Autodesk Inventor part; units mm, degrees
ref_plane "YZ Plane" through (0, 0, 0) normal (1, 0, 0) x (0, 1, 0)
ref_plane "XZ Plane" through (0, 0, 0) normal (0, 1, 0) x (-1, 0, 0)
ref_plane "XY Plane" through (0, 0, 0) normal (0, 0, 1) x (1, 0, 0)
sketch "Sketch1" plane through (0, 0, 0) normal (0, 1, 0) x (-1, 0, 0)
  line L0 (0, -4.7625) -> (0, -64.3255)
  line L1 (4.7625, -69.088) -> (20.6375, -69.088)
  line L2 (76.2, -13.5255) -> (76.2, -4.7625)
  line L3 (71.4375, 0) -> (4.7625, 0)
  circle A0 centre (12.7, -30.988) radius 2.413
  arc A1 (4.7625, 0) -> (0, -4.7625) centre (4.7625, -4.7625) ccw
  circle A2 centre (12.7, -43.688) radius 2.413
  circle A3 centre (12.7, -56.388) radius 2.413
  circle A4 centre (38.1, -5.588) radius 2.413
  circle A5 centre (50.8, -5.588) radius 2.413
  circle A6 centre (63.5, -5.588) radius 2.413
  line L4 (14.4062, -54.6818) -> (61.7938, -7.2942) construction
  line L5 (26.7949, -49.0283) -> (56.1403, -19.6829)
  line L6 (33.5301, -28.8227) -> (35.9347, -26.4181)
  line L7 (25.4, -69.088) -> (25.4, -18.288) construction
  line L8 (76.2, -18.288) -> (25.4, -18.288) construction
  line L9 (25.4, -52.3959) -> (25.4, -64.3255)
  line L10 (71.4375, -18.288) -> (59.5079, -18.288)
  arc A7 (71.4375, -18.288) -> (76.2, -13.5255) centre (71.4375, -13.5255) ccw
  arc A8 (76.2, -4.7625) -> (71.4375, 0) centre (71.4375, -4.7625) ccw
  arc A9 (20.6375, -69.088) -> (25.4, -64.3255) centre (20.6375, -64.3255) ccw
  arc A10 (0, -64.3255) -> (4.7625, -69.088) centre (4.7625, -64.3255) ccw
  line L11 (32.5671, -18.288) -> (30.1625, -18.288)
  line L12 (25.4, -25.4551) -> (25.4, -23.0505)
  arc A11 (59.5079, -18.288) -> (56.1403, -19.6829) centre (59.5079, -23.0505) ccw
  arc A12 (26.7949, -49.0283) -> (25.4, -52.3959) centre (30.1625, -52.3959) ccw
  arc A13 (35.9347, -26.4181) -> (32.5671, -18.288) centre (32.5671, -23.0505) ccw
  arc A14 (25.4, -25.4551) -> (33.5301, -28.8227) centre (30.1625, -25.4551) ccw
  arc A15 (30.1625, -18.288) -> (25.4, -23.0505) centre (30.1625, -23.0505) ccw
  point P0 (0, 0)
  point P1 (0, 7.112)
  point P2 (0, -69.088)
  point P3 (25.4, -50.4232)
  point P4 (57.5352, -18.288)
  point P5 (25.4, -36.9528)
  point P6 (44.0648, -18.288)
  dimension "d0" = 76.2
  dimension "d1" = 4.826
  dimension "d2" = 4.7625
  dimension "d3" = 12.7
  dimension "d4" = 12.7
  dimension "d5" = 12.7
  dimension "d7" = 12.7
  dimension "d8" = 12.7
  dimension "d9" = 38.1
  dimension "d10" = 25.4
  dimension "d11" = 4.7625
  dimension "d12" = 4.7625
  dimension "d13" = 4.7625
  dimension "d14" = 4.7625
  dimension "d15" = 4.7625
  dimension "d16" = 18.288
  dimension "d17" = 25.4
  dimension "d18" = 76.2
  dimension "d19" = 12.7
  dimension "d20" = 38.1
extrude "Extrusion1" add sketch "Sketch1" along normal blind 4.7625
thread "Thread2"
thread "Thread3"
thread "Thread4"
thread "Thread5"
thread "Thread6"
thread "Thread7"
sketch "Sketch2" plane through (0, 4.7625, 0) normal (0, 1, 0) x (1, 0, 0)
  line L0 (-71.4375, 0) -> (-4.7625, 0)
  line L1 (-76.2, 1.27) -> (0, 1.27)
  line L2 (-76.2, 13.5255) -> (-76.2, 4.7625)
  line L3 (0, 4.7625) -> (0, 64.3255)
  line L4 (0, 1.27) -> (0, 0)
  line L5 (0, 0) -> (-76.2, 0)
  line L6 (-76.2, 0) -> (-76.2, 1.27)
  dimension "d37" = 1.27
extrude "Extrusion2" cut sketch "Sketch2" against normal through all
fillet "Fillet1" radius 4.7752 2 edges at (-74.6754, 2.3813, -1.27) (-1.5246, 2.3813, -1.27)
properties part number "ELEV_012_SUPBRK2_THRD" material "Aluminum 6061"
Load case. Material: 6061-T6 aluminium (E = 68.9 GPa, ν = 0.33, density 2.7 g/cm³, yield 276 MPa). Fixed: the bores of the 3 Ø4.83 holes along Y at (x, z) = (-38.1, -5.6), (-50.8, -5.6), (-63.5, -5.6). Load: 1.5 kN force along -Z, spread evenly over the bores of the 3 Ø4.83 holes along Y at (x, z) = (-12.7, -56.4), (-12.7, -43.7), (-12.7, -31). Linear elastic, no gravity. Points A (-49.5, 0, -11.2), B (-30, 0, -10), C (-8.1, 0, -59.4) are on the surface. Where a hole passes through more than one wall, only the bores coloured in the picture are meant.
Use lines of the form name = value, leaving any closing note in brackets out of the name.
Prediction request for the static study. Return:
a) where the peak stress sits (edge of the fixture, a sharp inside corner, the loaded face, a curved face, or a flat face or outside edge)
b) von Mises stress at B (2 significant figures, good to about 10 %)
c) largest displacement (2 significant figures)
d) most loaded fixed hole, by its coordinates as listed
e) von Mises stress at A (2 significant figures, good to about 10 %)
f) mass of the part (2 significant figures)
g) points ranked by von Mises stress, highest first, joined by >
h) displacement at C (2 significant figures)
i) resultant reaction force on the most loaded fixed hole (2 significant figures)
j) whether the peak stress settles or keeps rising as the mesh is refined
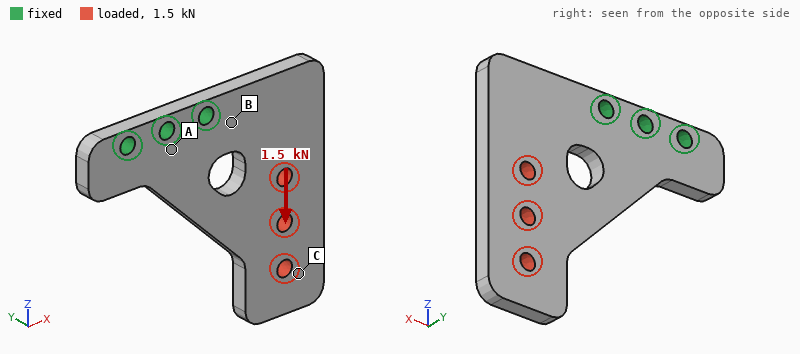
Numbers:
where the peak stress sits = edge of the fixture
von Mises stress at B = 47 MPa
largest displacement = 0.12 mm
most loaded fixed hole, by its coordinates as listed = (-38.1, -5.6)
von Mises stress at A = 21 MPa
mass of the part = 37 g
points ranked by von Mises stress, highest first, joined by > = B > A > C
displacement at C = 0.10 mm
resultant reaction force on the most loaded fixed hole = 3.1 kN
whether the peak stress settles or keeps rising as the mesh is refined = keeps rising
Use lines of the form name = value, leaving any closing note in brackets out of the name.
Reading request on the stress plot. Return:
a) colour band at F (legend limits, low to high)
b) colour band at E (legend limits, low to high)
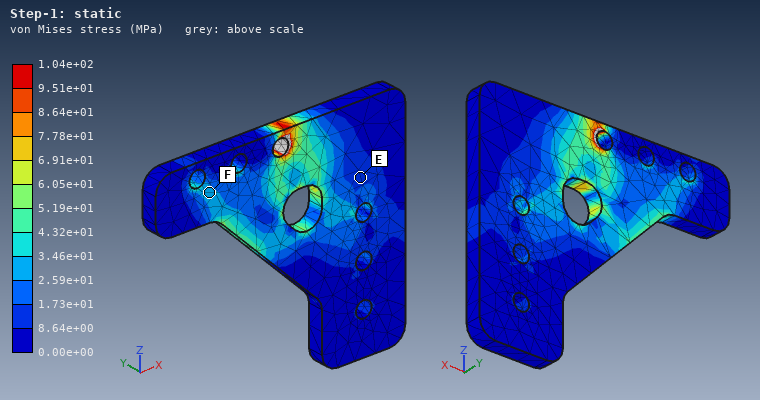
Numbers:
colour band at F = 2.59e+01 to 3.46e+01 MPa
colour band at E = 8.64e+00 to 1.73e+01 MPa
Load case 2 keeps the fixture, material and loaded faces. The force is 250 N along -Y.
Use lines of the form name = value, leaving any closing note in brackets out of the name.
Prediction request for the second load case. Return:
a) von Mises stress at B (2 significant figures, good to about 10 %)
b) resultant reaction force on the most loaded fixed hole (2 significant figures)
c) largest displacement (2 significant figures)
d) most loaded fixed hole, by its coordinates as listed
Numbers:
von Mises stress at B = 78 MPa
resultant reaction force on the most loaded fixed hole = 440 N
largest displacement = 0.81 mm
most loaded fixed hole, by its coordinates as listed = (-38.1, -5.6)
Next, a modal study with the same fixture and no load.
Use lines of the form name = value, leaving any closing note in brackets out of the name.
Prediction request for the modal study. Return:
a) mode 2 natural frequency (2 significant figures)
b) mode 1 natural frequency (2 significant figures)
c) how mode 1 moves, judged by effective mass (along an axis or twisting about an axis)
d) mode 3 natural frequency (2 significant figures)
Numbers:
mode 2 natural frequency = 2500 Hz
mode 1 natural frequency = 860 Hz
how mode 1 moves, judged by effective mass = along Y
mode 3 natural frequency = 3800 Hz
